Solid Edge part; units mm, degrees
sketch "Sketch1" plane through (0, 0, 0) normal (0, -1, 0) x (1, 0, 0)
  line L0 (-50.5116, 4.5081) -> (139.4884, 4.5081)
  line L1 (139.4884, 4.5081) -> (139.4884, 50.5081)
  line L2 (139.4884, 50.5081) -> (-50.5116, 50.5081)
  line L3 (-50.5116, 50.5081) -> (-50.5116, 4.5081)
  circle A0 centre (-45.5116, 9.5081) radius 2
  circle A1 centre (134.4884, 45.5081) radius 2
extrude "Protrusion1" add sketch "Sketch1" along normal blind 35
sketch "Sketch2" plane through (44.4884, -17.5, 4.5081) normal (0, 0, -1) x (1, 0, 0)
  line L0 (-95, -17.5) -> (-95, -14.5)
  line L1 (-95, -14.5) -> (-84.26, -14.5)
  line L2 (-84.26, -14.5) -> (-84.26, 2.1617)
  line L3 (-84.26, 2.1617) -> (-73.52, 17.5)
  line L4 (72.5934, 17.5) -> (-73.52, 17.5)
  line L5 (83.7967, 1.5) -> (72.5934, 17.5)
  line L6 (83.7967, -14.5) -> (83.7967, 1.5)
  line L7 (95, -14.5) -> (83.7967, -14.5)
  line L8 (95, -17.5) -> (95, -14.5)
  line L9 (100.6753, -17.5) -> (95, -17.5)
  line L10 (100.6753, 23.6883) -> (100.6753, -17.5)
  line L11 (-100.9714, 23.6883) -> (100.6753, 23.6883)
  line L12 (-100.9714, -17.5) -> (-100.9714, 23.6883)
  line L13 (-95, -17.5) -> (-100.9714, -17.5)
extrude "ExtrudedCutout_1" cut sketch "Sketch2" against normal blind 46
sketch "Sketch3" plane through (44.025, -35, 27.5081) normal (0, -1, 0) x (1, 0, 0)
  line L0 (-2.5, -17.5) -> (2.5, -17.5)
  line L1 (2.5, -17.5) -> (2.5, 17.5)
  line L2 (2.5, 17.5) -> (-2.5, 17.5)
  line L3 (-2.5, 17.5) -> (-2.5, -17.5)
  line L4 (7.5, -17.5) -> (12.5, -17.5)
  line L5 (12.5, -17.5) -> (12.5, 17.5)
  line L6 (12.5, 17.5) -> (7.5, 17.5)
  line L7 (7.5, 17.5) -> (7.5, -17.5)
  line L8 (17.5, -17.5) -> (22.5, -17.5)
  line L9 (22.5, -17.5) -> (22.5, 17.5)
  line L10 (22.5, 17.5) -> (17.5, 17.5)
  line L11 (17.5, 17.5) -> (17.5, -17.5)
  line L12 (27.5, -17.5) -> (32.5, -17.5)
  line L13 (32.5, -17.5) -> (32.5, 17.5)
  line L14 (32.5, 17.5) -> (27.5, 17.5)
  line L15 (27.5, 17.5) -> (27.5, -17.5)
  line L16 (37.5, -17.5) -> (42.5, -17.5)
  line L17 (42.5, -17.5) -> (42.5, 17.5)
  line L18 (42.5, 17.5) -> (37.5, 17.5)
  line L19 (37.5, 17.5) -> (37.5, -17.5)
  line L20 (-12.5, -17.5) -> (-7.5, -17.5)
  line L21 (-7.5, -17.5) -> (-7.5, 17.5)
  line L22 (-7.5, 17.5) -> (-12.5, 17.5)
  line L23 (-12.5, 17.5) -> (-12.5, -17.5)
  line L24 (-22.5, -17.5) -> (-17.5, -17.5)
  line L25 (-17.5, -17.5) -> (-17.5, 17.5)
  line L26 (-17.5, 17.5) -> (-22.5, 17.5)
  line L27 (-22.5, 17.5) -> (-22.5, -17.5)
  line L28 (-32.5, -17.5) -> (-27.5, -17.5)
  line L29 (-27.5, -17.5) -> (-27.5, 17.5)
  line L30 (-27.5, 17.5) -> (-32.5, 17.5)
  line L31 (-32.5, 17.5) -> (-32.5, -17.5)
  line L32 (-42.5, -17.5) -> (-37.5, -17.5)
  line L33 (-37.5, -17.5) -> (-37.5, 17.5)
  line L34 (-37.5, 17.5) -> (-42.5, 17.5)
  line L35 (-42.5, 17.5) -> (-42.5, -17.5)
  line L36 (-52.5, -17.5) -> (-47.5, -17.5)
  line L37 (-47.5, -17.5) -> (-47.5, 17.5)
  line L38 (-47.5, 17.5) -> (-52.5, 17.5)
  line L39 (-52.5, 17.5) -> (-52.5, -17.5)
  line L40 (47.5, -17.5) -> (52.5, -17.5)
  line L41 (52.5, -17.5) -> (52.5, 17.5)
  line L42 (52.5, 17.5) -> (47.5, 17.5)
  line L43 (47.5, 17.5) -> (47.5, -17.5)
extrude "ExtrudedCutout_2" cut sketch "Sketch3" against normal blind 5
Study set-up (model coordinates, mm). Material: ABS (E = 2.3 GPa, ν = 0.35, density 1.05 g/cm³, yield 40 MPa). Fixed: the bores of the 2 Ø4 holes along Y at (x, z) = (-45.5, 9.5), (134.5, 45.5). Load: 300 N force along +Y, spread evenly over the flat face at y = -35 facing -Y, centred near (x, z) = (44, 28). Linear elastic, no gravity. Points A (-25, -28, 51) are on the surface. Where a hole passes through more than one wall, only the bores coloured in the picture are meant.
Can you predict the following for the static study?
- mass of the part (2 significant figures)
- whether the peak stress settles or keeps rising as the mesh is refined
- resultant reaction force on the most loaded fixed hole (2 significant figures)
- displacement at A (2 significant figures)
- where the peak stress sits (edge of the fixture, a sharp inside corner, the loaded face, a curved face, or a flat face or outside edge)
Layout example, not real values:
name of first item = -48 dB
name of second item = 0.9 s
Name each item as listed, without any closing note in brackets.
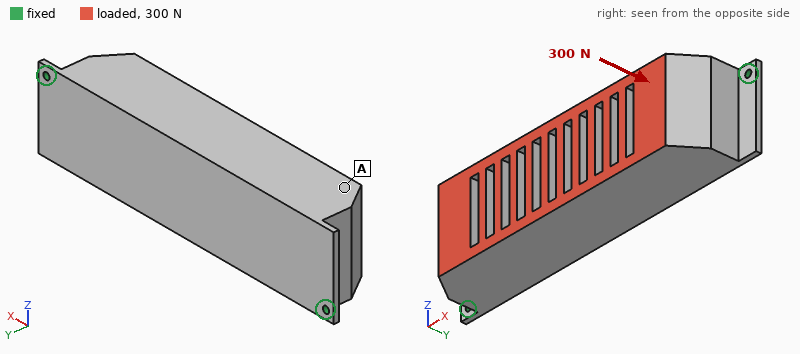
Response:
mass of the part = 270 g
whether the peak stress settles or keeps rising as the mesh is refined = keeps rising
resultant reaction force on the most loaded fixed hole = 200 N
displacement at A = 0.16 mm
where the peak stress sits = edge of the fixture
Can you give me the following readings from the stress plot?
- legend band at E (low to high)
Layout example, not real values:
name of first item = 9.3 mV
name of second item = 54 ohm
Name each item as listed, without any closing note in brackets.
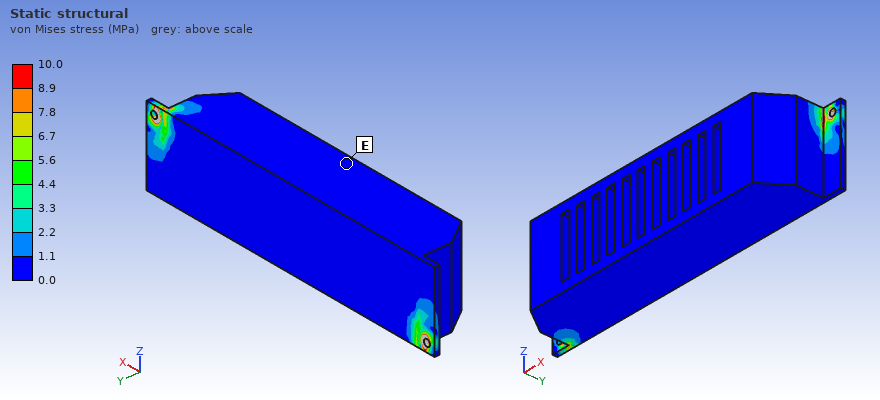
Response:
legend band at E = 0.0 to 1.1 MPa
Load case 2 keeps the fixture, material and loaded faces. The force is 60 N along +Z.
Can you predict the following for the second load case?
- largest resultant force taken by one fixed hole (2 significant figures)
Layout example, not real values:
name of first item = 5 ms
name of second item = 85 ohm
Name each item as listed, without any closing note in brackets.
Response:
largest resultant force taken by one fixed hole = 30 N
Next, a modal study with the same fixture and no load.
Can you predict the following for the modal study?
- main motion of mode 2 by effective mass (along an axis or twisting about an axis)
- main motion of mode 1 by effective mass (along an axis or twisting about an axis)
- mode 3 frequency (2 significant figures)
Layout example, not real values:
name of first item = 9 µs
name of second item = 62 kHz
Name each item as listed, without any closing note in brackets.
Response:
main motion of mode 2 by effective mass = along Y
main motion of mode 1 by effective mass = along Z
mode 3 frequency = 730 Hz
